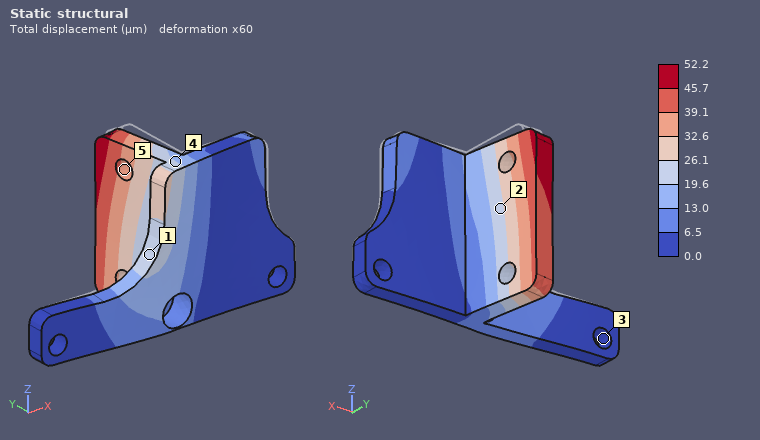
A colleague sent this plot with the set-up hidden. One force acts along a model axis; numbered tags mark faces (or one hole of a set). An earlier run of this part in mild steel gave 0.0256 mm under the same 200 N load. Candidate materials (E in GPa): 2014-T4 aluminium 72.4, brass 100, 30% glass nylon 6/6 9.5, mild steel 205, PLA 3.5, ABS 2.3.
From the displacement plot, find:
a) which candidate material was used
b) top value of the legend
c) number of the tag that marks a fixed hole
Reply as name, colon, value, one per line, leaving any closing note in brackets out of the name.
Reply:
which candidate material was used: brass
top value of the legend: 52.2 µm
number of the tag that marks a fixed hole: 3
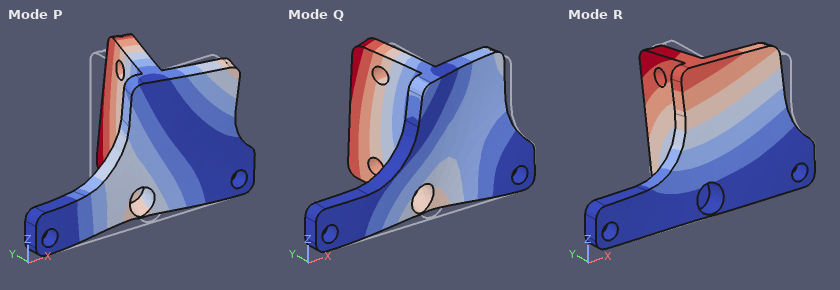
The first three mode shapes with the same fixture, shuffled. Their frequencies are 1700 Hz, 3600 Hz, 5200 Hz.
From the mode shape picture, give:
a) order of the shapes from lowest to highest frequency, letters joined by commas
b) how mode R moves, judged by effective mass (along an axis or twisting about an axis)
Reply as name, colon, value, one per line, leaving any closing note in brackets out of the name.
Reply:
order of the shapes from lowest to highest frequency, letters joined by commas: R, P, Q
how mode R moves, judged by effective mass: along Y
